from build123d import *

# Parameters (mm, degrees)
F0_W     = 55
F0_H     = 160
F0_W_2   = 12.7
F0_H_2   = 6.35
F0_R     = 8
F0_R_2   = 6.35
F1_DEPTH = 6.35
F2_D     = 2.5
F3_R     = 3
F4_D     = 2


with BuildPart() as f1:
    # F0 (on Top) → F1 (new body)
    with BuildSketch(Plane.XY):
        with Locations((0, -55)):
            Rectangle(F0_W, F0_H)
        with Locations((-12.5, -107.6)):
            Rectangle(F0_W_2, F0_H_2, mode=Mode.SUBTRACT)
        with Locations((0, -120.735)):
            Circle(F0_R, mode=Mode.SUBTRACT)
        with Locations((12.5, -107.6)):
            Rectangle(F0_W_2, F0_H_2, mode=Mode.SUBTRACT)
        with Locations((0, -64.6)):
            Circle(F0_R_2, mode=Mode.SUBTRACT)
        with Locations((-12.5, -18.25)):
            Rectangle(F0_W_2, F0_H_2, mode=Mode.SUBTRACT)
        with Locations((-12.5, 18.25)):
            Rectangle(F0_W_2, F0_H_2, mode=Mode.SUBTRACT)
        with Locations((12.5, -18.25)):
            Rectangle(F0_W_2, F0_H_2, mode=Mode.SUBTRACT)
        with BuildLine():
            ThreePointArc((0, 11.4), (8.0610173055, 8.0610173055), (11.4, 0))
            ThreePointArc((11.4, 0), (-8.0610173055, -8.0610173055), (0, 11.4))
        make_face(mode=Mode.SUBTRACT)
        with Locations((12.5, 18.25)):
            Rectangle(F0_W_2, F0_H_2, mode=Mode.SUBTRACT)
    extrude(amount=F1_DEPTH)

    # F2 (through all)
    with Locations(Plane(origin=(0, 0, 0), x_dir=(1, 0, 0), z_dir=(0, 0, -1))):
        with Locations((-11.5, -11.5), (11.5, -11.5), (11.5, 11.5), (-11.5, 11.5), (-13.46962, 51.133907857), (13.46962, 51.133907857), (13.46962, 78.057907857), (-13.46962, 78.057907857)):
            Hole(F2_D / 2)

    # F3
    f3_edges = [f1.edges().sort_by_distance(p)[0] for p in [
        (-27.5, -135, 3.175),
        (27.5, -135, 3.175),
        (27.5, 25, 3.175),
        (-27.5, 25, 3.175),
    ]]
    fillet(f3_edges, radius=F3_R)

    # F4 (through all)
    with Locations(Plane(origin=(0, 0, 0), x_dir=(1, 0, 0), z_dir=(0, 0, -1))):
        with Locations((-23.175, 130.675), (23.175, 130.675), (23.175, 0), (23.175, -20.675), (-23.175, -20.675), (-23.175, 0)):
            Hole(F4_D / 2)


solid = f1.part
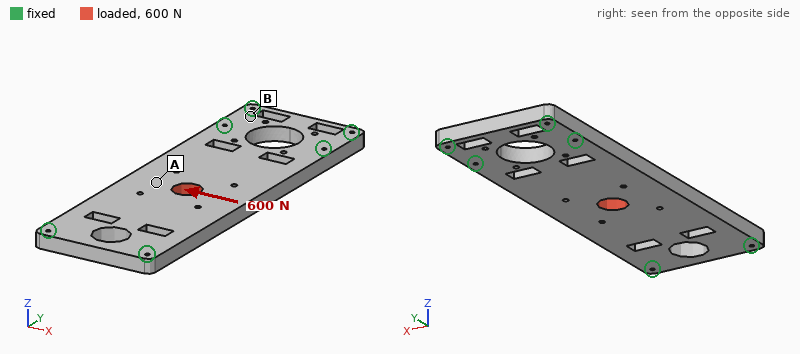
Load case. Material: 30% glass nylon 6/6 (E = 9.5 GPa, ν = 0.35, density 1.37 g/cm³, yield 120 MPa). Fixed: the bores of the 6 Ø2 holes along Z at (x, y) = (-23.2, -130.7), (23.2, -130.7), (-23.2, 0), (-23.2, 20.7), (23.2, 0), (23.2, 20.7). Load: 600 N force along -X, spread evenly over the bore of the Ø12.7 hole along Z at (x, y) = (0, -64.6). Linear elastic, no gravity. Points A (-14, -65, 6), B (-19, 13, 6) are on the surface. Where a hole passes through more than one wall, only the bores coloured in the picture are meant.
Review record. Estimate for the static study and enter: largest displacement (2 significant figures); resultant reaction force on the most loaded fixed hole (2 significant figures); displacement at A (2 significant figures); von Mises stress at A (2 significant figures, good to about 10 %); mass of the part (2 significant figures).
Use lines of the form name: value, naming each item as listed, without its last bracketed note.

largest displacement: 41 µm
resultant reaction force on the most loaded fixed hole: 240 N
displacement at A: 39 µm
von Mises stress at A: 2.0 MPa
mass of the part: 65 g
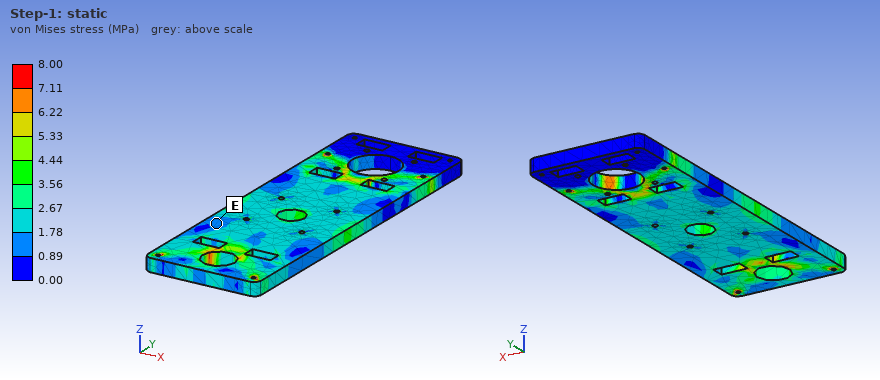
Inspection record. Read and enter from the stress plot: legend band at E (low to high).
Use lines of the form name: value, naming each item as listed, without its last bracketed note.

legend band at E: 0.89 to 1.78 MPa
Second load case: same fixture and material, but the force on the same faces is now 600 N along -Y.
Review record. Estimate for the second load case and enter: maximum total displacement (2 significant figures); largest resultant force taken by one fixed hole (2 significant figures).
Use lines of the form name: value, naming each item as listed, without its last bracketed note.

maximum total displacement: 12 µm
largest resultant force taken by one fixed hole: 150 N
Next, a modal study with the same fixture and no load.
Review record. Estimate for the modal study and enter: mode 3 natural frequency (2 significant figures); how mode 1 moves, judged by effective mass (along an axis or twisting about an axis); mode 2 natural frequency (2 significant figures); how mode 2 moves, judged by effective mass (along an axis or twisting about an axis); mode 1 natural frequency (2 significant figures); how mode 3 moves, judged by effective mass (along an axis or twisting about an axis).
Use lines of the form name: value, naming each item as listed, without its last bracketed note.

mode 3 natural frequency: 2300 Hz
how mode 1 moves, judged by effective mass: along Z
mode 2 natural frequency: 1600 Hz
how mode 2 moves, judged by effective mass: twisting about Y
mode 1 natural frequency: 800 Hz
how mode 3 moves, judged by effective mass: twisting about X
